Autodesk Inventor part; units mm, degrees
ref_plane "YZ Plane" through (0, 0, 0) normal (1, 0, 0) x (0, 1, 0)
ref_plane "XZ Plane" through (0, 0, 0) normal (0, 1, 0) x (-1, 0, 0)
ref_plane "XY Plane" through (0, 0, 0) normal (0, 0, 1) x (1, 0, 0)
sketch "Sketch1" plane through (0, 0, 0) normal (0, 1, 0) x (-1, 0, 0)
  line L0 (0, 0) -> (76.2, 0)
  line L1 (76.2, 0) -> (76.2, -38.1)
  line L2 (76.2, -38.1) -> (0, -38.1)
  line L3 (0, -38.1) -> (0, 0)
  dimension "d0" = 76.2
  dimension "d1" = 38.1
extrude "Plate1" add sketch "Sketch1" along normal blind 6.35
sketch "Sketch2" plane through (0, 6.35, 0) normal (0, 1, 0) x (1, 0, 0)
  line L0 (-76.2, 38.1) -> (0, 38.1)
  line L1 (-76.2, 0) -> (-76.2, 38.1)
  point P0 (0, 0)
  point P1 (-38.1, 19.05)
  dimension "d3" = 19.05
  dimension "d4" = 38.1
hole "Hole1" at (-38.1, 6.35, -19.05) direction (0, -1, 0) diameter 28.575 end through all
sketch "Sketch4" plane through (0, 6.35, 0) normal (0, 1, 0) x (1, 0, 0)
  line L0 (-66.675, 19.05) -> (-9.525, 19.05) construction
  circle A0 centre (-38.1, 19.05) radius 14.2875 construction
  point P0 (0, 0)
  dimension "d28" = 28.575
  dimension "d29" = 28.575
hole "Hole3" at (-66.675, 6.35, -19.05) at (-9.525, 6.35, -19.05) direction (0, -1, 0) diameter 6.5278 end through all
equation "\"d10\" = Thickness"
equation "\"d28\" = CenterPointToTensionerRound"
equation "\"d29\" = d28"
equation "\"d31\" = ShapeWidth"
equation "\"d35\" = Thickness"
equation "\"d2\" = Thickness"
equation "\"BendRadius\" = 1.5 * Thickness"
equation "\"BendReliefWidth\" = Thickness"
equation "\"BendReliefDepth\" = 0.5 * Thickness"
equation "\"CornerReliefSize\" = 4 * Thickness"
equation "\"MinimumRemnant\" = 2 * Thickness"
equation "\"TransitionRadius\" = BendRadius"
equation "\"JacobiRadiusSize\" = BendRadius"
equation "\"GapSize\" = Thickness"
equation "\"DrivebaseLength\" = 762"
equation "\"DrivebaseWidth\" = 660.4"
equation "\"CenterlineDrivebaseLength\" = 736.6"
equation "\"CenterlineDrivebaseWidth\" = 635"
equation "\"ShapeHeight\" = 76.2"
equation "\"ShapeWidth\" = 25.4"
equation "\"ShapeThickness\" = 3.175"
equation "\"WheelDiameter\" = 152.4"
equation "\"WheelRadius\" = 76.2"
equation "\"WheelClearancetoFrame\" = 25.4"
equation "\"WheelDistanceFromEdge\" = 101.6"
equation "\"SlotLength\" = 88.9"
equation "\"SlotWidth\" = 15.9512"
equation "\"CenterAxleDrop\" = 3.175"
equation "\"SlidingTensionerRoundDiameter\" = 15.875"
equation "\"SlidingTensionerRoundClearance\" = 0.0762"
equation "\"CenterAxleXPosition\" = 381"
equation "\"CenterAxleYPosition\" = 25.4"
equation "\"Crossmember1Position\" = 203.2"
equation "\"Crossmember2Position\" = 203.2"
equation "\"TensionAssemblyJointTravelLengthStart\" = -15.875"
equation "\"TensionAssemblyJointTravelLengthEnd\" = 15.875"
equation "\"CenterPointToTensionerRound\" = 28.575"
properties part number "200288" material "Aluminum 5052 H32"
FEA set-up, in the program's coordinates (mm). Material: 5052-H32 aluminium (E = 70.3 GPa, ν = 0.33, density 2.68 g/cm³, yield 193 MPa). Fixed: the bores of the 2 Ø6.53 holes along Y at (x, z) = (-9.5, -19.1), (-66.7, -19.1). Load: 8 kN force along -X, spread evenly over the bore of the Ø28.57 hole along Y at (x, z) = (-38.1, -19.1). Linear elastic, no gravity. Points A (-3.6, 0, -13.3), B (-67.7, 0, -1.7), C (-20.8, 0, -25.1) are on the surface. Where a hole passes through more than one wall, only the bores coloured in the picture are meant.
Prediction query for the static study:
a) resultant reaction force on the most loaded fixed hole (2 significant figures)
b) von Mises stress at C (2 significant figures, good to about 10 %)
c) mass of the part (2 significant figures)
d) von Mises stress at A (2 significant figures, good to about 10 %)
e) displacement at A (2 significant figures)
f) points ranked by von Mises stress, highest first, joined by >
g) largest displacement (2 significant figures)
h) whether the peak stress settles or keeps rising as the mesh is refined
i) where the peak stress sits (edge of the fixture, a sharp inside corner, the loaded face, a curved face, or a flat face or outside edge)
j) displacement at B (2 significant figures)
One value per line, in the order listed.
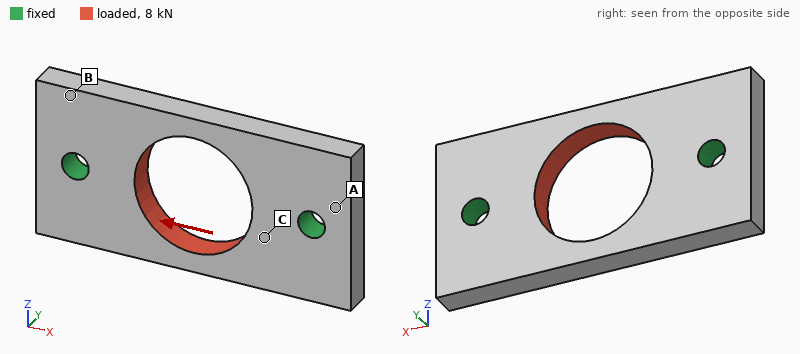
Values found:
4.0 kN
31 MPa
37 g
18 MPa
2.4 µm
C > A > B
14 µm
keeps rising
edge of the fixture
8.1 µm
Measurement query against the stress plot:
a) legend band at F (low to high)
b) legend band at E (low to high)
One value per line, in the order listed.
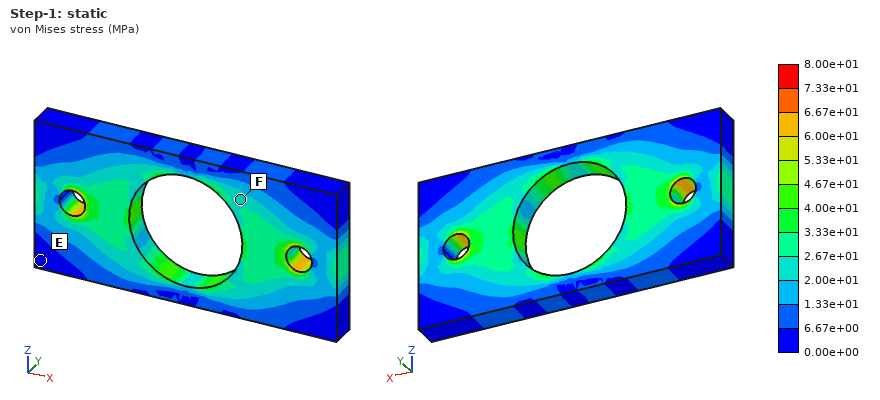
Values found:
2.00e+01 to 2.67e+01 MPa
0.00e+00 to 6.67e+00 MPa
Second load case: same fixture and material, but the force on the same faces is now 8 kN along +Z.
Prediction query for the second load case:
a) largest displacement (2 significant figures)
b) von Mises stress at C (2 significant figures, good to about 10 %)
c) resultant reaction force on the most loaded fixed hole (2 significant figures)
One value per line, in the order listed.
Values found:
37 µm
43 MPa
4.0 kN
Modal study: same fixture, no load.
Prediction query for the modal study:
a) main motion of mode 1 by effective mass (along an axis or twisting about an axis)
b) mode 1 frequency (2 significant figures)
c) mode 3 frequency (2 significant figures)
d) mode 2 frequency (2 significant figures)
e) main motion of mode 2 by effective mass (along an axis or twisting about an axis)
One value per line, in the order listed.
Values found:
twisting about X
8600 Hz
14 kHz
9500 Hz
along Y
